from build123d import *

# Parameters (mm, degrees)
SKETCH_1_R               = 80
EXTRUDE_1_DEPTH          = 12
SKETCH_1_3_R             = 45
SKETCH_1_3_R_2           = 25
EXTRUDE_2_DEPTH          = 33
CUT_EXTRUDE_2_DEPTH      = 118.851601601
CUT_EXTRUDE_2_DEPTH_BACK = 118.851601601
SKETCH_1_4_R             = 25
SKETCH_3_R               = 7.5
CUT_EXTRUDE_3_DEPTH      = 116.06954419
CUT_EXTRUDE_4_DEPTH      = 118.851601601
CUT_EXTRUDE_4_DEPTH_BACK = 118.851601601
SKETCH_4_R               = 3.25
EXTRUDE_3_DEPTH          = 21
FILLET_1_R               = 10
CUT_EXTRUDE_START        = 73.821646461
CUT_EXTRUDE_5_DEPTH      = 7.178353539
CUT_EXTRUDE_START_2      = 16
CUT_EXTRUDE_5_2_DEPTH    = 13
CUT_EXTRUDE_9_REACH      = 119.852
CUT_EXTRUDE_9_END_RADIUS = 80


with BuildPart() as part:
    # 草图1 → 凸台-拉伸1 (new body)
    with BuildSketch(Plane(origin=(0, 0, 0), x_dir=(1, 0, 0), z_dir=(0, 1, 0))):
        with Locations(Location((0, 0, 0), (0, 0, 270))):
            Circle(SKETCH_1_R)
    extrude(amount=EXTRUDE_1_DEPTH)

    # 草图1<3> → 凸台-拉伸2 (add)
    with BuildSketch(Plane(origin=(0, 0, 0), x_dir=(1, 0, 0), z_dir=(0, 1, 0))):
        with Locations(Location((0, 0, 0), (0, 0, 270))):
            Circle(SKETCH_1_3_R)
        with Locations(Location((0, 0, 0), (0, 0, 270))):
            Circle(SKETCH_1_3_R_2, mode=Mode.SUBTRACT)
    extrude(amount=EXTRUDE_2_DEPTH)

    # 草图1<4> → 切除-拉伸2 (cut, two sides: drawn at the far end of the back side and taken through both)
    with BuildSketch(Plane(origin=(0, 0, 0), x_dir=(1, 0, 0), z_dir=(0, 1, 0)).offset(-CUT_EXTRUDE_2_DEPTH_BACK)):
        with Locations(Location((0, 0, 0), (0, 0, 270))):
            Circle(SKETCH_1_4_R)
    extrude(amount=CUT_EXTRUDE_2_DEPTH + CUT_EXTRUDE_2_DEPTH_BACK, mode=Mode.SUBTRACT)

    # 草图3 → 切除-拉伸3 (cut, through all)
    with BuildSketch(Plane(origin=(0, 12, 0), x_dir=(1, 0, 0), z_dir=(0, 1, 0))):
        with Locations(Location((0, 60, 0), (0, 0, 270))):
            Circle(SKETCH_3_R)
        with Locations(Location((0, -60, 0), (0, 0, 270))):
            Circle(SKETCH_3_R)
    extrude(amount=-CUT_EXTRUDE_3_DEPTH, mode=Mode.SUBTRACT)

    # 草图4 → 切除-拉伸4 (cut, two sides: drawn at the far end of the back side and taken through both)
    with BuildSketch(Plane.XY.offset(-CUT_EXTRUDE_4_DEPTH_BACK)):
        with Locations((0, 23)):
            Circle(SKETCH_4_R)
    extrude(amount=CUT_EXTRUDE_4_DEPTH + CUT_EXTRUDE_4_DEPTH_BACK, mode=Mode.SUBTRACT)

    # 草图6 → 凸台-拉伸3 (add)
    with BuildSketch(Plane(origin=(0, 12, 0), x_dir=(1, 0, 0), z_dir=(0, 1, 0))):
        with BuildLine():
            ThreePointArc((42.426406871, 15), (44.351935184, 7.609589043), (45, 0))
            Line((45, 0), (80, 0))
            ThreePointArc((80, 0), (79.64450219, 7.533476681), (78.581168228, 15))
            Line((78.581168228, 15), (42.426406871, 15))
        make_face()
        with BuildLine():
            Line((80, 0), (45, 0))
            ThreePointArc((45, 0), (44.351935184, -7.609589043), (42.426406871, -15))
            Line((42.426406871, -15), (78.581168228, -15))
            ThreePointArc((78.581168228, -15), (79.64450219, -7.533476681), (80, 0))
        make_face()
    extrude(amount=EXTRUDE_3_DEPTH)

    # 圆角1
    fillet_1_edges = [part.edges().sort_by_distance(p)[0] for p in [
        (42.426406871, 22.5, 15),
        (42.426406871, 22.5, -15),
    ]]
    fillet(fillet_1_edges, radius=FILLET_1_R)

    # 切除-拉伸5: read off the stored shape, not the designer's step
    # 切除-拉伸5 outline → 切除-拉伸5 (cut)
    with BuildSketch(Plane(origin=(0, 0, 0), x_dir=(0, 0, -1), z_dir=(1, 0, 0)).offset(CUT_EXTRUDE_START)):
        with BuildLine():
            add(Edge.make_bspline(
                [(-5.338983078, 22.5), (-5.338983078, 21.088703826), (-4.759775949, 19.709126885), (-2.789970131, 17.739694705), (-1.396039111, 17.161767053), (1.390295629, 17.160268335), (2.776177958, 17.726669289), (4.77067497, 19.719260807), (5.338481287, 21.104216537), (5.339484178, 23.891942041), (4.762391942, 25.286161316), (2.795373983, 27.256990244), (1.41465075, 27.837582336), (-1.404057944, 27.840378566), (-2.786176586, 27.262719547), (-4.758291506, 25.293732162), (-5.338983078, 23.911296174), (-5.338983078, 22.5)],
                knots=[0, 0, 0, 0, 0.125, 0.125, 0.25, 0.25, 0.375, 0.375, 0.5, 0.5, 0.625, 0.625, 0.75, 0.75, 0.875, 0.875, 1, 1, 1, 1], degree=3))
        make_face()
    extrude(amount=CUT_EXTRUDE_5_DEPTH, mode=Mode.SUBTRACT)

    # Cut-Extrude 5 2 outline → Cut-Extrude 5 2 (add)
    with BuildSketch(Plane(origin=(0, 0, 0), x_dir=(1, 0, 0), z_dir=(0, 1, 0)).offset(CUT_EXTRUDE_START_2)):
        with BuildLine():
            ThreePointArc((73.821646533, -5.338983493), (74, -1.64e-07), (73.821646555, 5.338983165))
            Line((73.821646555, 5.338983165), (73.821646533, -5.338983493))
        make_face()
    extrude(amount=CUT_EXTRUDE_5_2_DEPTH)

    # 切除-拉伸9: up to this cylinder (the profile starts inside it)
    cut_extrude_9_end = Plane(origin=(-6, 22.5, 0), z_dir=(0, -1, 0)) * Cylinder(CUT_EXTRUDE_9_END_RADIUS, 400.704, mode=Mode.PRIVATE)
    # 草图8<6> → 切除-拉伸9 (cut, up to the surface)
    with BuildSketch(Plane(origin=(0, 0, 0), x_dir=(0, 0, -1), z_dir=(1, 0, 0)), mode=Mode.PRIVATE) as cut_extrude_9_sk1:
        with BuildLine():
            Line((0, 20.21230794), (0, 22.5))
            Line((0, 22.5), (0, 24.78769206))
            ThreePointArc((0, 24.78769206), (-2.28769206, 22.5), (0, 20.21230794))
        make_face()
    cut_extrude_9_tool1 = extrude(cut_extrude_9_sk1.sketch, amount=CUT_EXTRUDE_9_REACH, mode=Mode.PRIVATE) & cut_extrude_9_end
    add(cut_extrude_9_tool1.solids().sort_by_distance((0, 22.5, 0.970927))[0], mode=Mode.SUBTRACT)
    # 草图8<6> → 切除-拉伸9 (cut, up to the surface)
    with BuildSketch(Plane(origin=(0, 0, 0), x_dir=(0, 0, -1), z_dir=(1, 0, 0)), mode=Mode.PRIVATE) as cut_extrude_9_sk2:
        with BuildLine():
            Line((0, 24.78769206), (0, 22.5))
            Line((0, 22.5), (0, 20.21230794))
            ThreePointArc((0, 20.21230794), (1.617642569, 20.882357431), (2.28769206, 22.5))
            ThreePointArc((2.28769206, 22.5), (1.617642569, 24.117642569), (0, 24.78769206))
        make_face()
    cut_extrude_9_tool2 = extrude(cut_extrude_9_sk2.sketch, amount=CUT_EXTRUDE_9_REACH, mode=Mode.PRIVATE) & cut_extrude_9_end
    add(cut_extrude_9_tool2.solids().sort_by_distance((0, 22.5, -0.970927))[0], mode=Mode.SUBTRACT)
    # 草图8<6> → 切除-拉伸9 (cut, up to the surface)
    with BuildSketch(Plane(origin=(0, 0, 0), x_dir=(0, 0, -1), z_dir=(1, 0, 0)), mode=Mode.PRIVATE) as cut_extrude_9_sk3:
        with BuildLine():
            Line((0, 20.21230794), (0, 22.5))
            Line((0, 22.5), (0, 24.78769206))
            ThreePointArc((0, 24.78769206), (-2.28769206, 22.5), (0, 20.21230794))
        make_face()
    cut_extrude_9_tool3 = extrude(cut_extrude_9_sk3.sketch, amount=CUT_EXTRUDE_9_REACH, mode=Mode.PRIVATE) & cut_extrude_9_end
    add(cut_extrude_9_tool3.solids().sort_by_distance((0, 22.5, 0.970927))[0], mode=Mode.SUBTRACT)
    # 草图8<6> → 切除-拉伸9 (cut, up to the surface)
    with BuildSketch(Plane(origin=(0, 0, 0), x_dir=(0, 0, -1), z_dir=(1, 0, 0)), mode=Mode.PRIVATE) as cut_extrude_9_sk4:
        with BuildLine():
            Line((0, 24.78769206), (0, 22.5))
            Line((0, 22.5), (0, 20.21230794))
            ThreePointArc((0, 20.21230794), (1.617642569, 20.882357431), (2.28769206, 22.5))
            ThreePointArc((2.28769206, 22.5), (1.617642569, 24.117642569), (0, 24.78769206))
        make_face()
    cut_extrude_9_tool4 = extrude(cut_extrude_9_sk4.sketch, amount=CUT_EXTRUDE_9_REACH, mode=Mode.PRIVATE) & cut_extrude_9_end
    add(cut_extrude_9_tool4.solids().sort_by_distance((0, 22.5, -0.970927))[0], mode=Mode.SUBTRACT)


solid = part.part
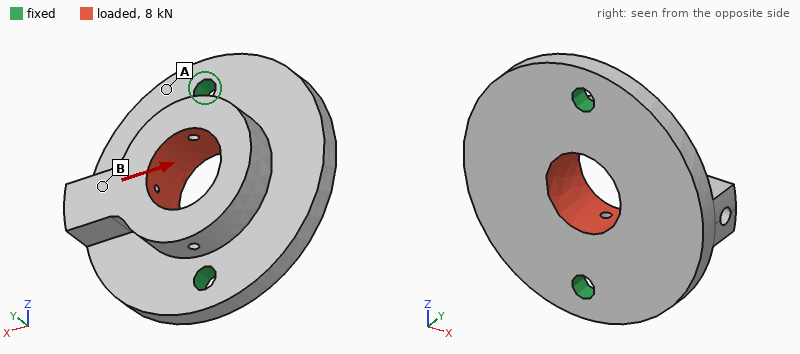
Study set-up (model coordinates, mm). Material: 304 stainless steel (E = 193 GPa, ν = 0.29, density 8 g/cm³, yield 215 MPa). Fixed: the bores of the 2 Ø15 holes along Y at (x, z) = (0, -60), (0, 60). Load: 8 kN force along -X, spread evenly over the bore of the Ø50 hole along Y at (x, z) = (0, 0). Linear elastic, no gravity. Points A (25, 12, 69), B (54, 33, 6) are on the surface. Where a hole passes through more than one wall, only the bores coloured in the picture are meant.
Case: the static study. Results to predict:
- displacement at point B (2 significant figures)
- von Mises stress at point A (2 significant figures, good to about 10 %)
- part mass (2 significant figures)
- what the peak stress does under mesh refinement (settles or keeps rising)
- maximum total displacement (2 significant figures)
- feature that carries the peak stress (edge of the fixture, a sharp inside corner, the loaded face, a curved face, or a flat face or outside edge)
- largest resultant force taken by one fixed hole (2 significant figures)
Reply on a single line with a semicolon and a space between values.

15 µm; 9.0 MPa; 2.6 kg; keeps rising; 20 µm; edge of the fixture; 4.0 kN
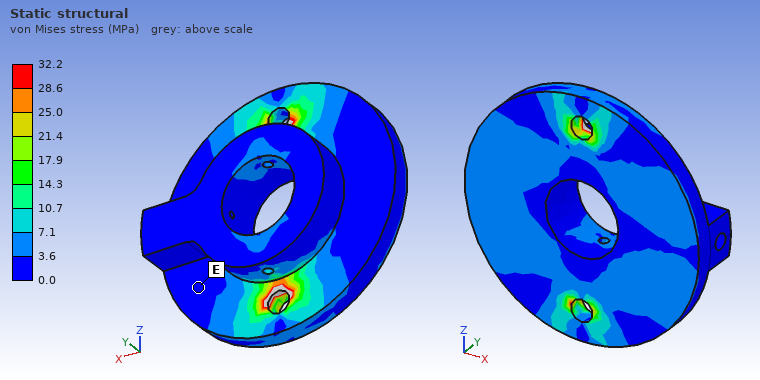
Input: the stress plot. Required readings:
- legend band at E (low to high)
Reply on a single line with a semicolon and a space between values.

0.0 to 3.6 MPa
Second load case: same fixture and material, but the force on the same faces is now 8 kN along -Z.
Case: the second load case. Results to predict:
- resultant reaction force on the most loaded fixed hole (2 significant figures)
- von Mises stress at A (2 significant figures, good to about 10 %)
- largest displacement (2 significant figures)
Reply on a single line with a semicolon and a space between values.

4.1 kN; 1.4 MPa; 1.9 µm
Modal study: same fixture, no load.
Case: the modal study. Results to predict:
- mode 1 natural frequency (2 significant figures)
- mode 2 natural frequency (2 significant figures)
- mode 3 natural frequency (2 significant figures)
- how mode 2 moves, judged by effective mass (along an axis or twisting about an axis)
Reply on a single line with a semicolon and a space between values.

1400 Hz; 2700 Hz; 5100 Hz; along Y
